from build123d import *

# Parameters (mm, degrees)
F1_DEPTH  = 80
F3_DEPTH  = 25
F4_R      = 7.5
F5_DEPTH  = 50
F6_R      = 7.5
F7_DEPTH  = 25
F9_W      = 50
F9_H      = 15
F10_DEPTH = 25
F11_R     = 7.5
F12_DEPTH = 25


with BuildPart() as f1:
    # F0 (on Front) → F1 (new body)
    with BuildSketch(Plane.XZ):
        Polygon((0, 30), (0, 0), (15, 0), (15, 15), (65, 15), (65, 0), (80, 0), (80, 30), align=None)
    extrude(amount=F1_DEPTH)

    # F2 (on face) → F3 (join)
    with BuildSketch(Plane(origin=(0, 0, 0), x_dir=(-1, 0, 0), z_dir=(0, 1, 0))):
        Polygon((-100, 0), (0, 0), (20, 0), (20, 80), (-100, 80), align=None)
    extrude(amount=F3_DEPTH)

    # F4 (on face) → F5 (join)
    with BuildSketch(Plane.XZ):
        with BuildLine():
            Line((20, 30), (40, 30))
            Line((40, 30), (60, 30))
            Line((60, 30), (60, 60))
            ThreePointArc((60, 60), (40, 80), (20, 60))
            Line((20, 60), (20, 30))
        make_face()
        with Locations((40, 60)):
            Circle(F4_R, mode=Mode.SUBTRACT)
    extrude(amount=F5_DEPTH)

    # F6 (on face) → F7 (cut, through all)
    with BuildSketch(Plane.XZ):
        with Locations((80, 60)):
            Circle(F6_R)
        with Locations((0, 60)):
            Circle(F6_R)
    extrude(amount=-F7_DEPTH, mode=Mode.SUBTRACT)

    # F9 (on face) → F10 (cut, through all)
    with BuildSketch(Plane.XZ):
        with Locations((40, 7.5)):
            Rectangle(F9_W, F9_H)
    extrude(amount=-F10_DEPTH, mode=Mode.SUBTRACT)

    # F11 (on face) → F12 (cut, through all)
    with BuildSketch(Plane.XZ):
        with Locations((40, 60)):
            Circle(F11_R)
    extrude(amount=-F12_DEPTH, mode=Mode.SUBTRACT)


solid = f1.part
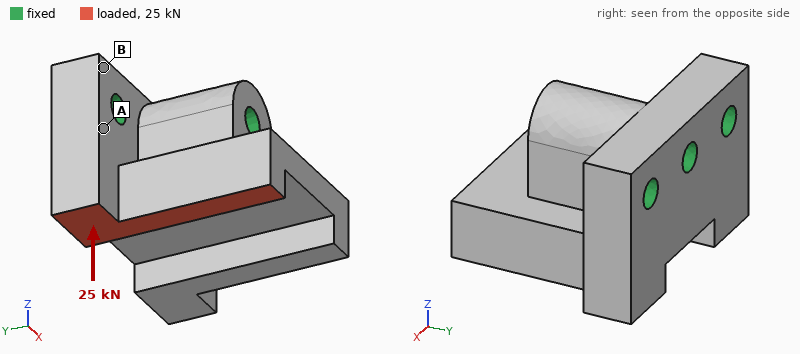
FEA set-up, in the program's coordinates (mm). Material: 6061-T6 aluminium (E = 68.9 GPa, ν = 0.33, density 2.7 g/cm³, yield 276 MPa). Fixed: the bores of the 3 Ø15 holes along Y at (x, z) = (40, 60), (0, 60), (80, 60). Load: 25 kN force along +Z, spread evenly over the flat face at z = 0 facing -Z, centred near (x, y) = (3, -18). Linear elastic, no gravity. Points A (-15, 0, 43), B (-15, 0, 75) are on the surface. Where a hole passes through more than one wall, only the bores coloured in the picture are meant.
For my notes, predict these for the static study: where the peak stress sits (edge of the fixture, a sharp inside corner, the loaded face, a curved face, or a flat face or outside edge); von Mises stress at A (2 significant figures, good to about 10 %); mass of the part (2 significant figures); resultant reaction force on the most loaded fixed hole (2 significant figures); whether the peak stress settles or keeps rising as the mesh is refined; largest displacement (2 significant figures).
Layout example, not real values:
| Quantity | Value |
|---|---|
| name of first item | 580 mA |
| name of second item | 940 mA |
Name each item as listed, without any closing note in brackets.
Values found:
| Quantity | Value |
|---|---|
| where the peak stress sits | a sharp inside corner |
| von Mises stress at A | 20 MPa |
| mass of the part | 1.1 kg |
| resultant reaction force on the most loaded fixed hole | 16 kN |
| whether the peak stress settles or keeps rising as the mesh is refined | keeps rising |
| largest displacement | 0.16 mm |
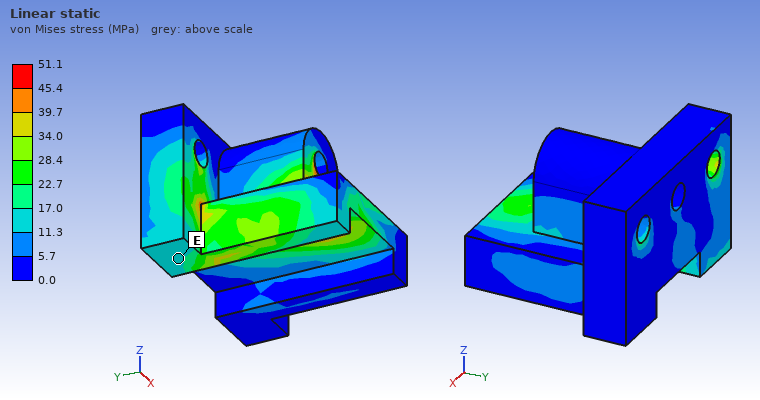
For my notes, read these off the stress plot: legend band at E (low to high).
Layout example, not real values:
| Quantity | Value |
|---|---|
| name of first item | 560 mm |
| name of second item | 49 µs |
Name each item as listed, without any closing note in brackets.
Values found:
| Quantity | Value |
|---|---|
| legend band at E | 11.3 to 17.0 MPa |
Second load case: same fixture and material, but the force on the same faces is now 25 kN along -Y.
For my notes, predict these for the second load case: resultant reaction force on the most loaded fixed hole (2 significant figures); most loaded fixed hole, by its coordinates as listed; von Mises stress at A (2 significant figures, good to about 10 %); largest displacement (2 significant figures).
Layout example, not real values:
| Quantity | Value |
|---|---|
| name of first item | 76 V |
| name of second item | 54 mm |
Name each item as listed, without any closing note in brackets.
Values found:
| Quantity | Value |
|---|---|
| resultant reaction force on the most loaded fixed hole | 20 kN |
| most loaded fixed hole, by its coordinates as listed | (40, 60) |
| von Mises stress at A | 37 MPa |
| largest displacement | 0.14 mm |
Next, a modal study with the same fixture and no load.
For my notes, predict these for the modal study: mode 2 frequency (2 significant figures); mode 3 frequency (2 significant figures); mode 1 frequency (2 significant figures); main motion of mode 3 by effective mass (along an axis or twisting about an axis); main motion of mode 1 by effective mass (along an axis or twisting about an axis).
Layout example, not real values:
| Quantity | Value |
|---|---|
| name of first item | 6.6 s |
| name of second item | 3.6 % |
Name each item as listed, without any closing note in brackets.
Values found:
| Quantity | Value |
|---|---|
| mode 2 frequency | 5800 Hz |
| mode 3 frequency | 6700 Hz |
| mode 1 frequency | 4700 Hz |
| main motion of mode 3 by effective mass | twisting about Z |
| main motion of mode 1 by effective mass | along X |
